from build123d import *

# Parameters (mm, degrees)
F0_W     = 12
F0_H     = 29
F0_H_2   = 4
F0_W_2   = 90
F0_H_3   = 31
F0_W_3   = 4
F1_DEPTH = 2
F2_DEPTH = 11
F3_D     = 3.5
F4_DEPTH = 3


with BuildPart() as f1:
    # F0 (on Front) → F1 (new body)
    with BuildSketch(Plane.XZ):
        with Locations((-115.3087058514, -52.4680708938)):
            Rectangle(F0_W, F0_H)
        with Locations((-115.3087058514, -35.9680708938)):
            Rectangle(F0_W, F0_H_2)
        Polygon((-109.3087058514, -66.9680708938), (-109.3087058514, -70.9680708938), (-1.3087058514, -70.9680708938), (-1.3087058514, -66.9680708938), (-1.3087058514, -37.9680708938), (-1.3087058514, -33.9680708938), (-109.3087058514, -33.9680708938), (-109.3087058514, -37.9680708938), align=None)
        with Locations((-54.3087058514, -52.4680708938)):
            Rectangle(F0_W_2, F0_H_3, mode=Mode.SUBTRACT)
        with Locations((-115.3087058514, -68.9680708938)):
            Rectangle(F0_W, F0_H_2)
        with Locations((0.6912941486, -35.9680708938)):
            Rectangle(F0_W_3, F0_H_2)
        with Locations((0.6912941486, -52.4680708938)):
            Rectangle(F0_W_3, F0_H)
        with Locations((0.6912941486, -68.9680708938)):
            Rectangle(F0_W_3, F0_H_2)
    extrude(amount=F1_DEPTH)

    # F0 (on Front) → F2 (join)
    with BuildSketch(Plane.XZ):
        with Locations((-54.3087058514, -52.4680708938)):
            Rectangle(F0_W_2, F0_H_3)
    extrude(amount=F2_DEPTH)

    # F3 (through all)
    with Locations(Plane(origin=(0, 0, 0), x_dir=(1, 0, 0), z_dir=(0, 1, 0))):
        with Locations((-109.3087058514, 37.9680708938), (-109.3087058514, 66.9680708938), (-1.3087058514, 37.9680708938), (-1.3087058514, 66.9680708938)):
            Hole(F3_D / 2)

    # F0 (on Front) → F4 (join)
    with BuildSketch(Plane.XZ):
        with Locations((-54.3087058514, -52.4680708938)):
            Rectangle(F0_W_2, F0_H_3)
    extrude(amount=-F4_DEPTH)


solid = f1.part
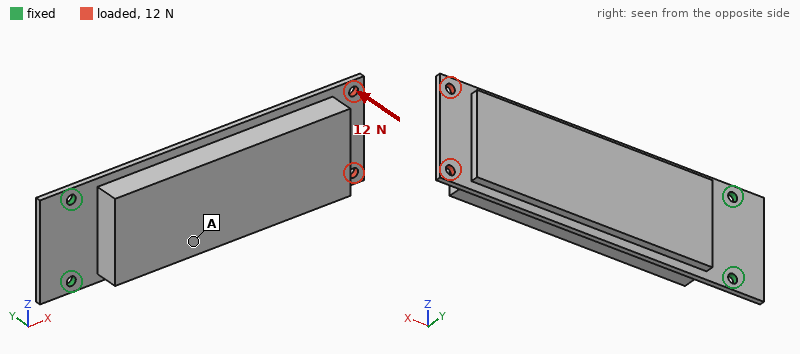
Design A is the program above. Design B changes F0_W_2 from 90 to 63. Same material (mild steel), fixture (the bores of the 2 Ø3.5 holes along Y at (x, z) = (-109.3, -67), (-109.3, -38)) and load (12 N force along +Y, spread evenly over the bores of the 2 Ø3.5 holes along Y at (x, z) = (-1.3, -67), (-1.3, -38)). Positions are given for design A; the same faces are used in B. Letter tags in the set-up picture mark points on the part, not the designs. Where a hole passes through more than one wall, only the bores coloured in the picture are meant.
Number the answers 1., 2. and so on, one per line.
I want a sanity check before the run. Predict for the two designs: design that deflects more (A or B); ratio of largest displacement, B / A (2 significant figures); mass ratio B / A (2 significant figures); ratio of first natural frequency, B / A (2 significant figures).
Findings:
1. B
2. 2.0
3. 0.76
4. 0.88
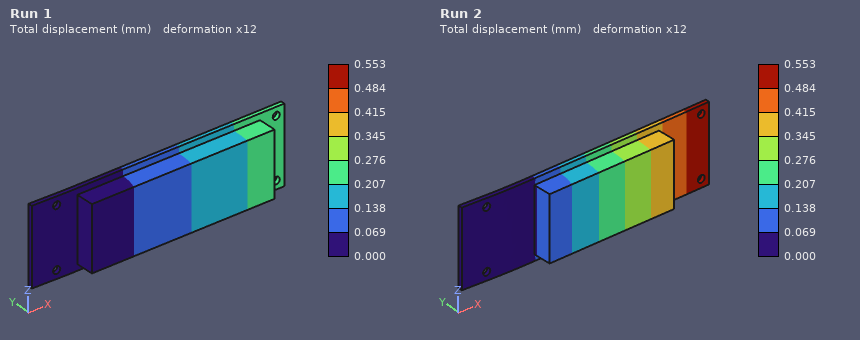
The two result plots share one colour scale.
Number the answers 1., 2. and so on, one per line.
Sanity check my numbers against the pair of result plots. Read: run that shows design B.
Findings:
1. Run 2
